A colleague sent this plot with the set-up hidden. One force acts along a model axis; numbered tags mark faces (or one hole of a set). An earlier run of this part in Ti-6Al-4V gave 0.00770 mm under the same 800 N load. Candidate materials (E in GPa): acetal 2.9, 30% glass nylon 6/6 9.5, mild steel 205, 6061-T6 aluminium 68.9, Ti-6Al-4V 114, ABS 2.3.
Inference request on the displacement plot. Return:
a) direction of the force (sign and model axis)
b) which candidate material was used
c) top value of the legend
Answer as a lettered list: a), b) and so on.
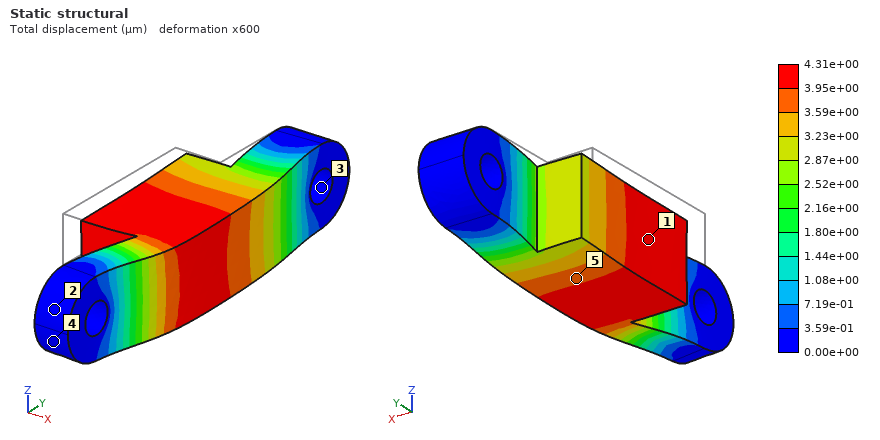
a) +X
b) mild steel
c) 4.31e+00 µm
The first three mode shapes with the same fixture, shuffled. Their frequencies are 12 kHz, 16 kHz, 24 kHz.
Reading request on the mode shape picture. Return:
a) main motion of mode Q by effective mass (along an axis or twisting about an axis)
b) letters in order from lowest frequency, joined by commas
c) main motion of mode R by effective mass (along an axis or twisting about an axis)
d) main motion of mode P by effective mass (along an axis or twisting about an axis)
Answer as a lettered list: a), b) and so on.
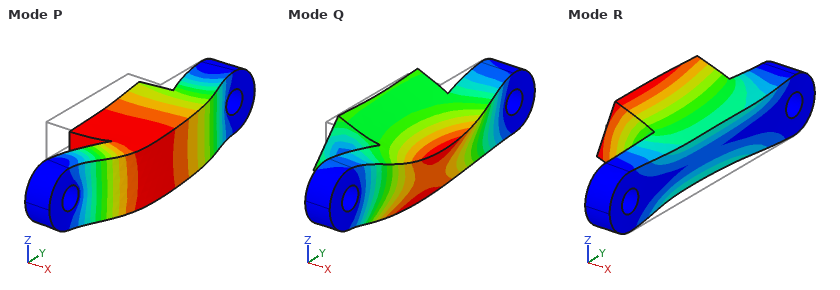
a) along Z
b) R, P, Q
c) along Z
d) along X
